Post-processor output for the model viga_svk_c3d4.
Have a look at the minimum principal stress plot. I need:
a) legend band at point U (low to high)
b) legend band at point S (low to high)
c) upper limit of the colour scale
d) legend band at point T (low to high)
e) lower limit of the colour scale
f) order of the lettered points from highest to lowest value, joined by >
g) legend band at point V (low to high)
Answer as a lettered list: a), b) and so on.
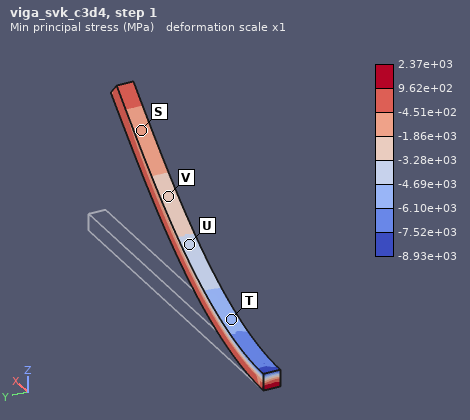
a) -4.69e+03 to -3.28e+03 MPa
b) -1.86e+03 to -4.51e+02 MPa
c) 2.37e+03 MPa
d) -6.10e+03 to -4.69e+03 MPa
e) -8.93e+03 MPa
f) S > V > U > T
g) -3.28e+03 to -1.86e+03 MPa
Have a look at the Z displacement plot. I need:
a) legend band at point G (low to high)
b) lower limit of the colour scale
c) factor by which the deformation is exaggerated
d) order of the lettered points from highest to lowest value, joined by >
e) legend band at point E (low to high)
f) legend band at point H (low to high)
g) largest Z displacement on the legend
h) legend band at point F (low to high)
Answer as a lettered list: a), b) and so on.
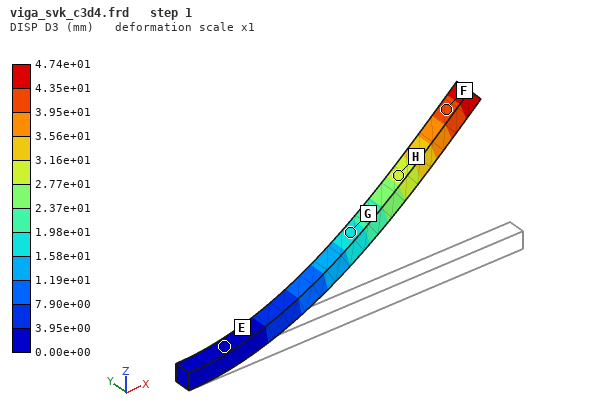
a) 1.58e+01 to 1.98e+01 mm
b) 0.00e+00 mm
c) 1
d) F > H > G > E
e) 0.00e+00 to 3.95e+00 mm
f) 2.77e+01 to 3.16e+01 mm
g) 4.74e+01 mm
h) 3.95e+01 to 4.35e+01 mm
